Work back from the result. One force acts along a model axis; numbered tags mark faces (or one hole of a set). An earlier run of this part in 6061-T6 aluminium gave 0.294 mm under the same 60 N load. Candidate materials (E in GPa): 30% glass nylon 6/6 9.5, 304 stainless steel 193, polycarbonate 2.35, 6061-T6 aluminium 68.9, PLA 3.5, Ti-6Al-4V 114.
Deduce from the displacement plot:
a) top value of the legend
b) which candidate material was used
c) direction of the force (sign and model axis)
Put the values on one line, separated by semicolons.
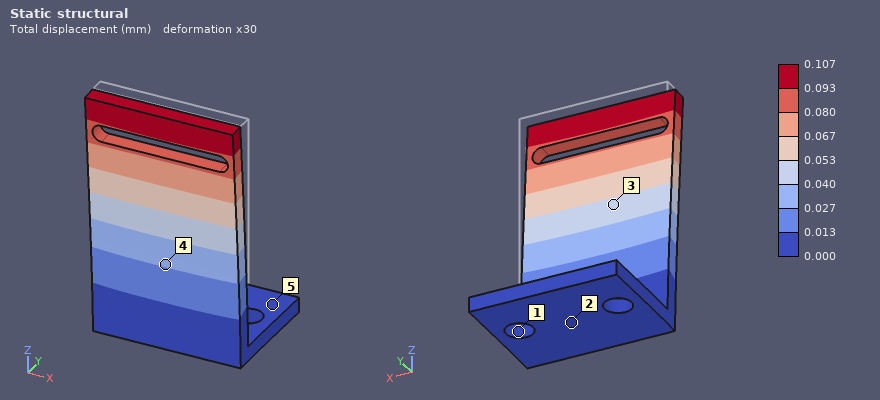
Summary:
0.107 mm; 304 stainless steel; -Y
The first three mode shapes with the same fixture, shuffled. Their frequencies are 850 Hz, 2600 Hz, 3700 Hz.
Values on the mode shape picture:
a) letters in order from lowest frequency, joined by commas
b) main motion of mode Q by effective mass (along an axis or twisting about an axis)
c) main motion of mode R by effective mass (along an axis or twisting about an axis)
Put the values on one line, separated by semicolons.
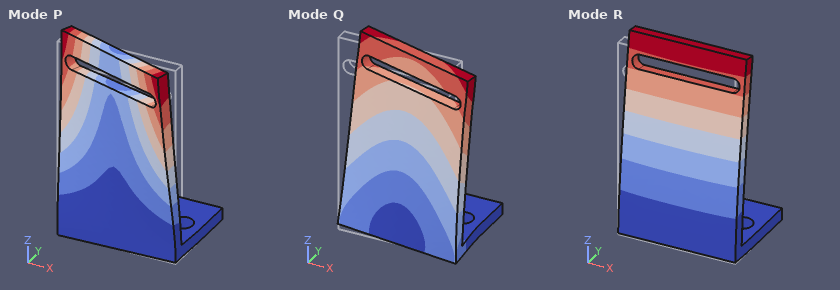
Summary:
R, Q, P; along X; along Y
